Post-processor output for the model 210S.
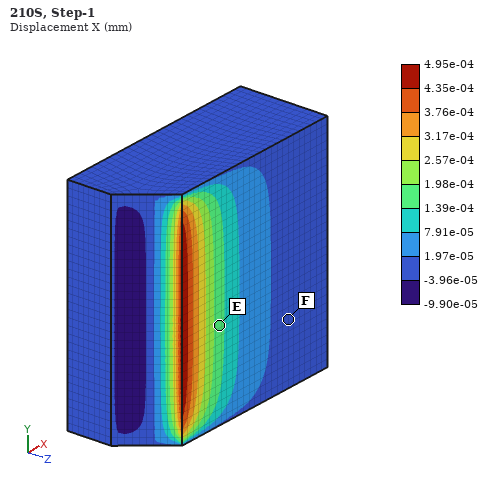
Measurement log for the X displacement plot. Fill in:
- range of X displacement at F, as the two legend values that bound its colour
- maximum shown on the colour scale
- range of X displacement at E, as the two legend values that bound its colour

-3.96e-05 to 1.97e-05 mm
4.95e-04 mm
1.39e-04 to 1.98e-04 mm
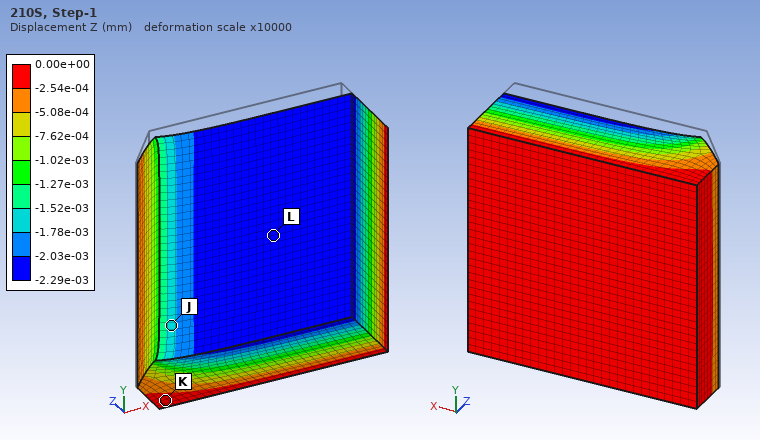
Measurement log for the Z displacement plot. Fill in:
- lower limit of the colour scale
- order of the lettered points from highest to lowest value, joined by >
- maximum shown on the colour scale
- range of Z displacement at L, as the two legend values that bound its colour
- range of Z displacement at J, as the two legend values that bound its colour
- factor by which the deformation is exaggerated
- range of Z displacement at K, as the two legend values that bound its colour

-2.29e-03 mm
K > J > L
0.00e+00 mm
-2.29e-03 to -2.03e-03 mm
-1.78e-03 to -1.52e-03 mm
10000
-2.54e-04 to 0.00e+00 mm
